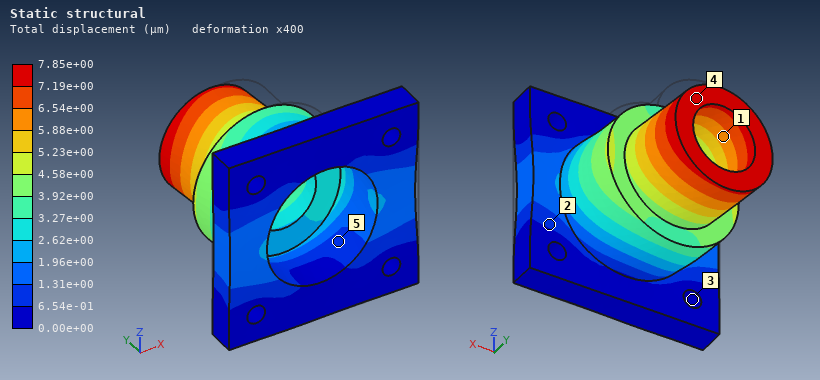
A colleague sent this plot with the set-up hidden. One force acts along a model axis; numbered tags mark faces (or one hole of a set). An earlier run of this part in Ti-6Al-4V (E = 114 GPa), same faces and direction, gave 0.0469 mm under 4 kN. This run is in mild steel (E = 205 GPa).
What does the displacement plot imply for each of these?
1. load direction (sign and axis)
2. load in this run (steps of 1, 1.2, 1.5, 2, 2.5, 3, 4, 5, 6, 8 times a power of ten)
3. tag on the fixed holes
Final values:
-X
1.2 kN
3
